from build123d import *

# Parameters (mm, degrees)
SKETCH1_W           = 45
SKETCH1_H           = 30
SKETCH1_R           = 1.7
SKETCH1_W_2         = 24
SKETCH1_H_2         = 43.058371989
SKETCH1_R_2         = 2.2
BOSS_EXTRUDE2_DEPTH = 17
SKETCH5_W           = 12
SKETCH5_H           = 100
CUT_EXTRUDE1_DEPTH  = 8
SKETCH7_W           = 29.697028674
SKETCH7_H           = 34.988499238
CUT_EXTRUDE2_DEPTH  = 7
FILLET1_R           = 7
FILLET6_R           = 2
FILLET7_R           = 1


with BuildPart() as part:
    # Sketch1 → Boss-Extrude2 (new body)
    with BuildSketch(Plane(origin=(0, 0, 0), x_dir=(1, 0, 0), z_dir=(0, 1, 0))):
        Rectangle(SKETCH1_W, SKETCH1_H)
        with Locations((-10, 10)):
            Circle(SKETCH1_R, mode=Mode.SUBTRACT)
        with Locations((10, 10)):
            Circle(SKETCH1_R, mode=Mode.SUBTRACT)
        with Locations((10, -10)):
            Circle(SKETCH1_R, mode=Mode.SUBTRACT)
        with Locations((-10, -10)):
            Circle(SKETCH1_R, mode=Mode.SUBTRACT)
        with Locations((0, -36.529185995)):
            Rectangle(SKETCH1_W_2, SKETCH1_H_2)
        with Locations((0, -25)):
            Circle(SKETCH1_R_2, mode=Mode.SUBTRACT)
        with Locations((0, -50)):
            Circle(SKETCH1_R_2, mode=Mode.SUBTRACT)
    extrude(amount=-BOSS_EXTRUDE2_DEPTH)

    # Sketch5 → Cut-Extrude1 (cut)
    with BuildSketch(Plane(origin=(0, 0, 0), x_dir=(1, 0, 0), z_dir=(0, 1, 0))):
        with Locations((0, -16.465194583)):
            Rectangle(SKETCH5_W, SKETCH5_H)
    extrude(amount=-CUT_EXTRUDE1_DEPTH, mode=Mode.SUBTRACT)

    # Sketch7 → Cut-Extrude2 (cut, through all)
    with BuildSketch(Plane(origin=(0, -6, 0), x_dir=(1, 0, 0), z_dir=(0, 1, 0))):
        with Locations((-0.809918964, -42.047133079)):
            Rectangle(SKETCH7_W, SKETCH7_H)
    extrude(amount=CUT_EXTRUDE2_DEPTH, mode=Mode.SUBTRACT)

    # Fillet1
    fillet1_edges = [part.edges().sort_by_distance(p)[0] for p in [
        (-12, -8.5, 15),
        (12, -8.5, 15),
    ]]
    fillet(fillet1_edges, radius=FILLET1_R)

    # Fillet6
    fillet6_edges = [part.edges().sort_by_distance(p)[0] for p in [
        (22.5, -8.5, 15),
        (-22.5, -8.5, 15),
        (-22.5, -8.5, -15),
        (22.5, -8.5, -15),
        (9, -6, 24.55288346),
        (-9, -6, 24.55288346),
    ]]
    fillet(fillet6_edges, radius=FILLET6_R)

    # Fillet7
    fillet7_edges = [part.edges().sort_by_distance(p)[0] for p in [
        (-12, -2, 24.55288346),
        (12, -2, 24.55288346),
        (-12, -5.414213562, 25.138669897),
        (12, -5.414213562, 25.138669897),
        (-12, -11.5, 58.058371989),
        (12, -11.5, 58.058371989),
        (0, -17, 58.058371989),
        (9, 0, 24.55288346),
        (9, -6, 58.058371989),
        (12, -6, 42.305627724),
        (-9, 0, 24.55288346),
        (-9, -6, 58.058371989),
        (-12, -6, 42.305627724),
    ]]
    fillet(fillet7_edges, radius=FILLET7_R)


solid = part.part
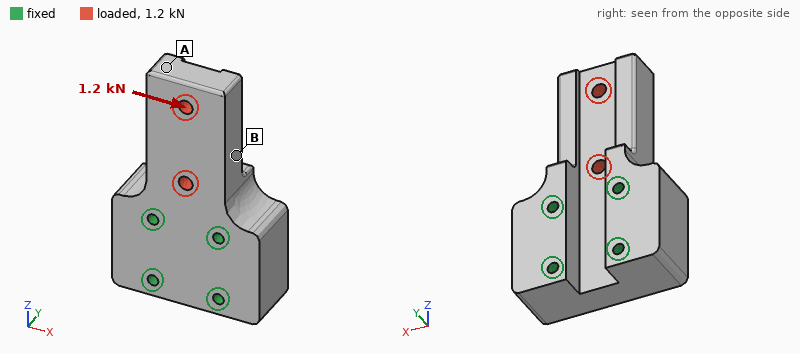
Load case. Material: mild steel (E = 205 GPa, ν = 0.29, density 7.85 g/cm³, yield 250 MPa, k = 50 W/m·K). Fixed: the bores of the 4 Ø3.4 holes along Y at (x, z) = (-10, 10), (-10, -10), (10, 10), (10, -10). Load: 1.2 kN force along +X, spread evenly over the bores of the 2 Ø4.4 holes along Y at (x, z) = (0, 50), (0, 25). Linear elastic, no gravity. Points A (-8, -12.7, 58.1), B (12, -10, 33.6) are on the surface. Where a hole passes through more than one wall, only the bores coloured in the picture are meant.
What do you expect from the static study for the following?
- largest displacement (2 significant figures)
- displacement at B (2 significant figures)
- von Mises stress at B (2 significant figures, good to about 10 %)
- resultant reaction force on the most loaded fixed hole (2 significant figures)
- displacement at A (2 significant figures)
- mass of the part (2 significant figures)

7.4 µm
3.2 µm
8.3 MPa
1.4 kN
7.0 µm
240 g
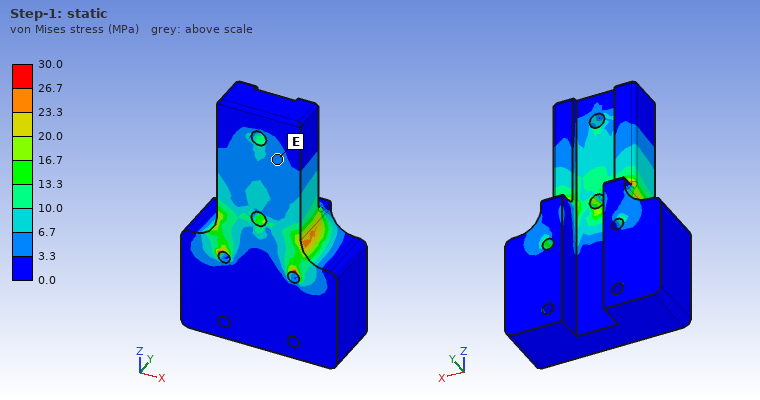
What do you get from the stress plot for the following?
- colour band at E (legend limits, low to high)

3.3 to 6.7 MPa
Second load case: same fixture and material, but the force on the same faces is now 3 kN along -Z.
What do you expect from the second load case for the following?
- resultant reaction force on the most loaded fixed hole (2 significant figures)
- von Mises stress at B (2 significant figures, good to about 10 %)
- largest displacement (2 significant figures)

1.3 kN
7.5 MPa
5.1 µm
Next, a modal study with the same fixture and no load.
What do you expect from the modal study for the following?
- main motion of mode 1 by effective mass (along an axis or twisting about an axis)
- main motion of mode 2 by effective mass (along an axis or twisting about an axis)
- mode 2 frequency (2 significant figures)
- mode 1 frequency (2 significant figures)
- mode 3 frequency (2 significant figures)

along Y
along X
8900 Hz
4900 Hz
13 kHz
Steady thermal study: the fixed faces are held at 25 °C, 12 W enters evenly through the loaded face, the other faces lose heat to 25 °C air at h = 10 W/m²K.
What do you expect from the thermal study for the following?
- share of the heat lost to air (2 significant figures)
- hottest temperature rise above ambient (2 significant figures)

4.8 %
26 K
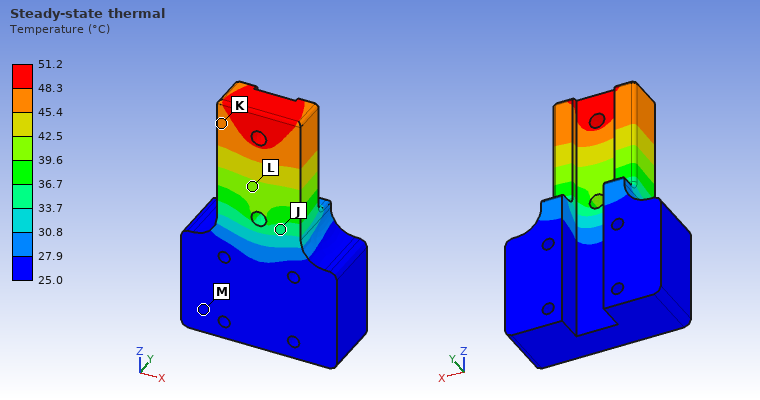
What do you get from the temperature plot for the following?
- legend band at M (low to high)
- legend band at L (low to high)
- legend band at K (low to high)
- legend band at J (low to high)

25.0 to 27.9 °C
39.6 to 42.5 °C
45.4 to 48.3 °C
33.7 to 36.7 °C
